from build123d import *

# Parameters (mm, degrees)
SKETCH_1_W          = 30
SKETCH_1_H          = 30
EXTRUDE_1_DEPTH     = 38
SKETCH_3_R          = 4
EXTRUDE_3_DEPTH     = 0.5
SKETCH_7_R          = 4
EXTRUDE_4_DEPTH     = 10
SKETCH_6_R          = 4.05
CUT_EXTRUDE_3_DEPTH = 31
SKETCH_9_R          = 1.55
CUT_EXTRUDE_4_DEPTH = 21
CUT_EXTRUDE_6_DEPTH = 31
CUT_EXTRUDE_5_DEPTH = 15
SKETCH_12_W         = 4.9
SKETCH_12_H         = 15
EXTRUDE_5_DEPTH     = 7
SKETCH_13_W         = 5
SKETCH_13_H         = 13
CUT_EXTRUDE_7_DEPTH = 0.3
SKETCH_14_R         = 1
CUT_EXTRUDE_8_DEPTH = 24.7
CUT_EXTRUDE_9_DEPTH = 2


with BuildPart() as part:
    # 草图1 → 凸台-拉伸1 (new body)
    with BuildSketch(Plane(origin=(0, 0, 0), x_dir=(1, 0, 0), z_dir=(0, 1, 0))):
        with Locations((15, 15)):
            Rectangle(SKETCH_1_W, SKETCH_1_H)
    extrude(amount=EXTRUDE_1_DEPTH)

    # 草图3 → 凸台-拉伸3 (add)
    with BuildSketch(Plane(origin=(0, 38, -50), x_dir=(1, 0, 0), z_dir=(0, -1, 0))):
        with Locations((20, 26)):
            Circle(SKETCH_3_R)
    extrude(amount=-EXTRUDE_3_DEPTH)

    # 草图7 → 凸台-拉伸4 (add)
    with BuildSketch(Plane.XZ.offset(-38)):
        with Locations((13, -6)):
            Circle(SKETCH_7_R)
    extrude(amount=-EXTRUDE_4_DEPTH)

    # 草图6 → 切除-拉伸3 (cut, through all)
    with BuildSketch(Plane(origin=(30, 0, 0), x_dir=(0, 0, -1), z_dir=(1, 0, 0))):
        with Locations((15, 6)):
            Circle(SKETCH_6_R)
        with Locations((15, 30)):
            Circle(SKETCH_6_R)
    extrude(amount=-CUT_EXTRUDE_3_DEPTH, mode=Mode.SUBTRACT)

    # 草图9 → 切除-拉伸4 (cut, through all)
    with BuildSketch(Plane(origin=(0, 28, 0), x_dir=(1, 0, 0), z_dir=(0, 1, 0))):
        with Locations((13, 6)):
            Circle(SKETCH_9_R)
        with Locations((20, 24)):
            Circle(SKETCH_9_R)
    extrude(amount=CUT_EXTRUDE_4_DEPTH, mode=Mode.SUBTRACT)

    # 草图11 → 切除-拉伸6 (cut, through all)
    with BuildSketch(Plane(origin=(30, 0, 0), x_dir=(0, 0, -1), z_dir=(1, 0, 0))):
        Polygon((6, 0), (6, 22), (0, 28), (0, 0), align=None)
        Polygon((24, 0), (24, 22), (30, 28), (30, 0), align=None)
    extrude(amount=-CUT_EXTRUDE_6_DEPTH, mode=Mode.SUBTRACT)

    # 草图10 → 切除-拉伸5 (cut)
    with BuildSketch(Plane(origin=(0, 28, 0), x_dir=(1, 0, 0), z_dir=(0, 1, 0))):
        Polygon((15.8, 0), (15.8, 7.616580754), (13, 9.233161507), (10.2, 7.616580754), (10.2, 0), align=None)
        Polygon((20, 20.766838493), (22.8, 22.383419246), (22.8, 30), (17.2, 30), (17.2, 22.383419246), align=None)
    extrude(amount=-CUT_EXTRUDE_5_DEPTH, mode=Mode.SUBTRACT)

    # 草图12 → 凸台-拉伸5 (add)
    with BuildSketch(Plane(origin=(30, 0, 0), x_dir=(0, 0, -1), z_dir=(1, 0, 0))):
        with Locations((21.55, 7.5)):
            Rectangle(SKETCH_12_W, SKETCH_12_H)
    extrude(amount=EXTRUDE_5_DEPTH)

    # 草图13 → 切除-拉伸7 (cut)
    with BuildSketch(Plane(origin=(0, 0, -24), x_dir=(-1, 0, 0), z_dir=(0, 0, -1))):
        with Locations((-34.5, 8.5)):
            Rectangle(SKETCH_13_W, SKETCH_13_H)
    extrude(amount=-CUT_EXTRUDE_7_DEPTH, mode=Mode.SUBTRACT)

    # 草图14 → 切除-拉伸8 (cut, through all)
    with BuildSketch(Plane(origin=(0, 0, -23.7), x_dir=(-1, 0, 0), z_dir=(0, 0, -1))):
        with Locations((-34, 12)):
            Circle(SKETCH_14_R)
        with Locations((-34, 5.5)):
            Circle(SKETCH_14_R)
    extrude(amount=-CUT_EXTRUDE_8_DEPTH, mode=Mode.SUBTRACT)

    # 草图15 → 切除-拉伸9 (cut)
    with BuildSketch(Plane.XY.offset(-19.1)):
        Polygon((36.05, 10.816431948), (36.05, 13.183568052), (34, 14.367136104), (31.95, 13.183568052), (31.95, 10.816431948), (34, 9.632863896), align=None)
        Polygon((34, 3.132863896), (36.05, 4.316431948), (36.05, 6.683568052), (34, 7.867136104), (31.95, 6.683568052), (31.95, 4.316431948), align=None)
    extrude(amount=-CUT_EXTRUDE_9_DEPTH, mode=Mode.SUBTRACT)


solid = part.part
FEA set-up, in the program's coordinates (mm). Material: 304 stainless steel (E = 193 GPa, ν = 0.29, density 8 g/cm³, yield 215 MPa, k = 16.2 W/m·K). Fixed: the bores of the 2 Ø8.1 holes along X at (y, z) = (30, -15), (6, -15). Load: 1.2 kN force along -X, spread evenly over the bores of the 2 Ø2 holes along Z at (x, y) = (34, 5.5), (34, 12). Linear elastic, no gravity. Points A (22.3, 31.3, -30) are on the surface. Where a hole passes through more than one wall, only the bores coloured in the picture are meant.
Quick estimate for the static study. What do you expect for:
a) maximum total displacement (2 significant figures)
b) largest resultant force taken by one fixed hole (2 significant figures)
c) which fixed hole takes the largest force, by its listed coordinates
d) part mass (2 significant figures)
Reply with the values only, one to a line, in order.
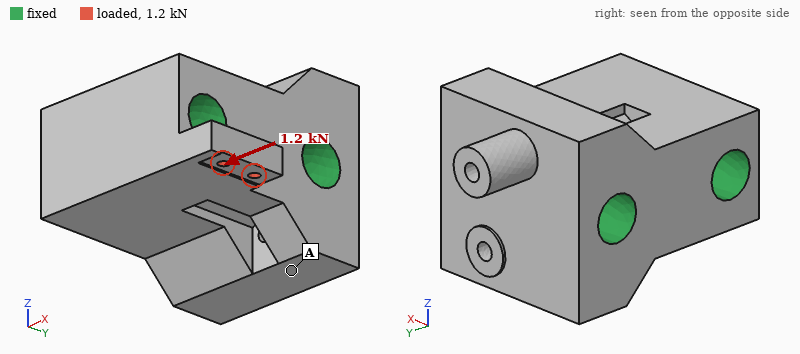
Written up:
3.6 µm
1.1 kN
(6, -15)
180 g
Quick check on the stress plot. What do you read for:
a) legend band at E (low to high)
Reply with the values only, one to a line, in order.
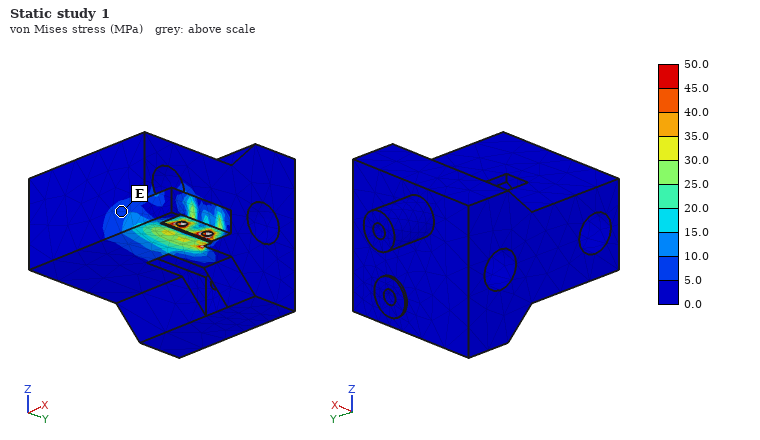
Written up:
5.0 to 10.0 MPa
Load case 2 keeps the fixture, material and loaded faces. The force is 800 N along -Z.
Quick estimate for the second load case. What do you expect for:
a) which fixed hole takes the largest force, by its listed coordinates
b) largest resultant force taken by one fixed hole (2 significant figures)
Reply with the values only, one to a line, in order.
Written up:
(6, -15)
750 N
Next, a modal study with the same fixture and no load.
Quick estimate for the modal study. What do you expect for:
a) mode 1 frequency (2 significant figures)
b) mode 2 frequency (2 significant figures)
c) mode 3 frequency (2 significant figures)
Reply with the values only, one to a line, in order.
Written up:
30 kHz
32 kHz
40 kHz
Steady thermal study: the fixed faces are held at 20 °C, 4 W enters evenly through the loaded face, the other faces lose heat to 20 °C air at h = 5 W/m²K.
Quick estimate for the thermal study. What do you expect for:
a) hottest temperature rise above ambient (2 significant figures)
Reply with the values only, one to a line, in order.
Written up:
39 K
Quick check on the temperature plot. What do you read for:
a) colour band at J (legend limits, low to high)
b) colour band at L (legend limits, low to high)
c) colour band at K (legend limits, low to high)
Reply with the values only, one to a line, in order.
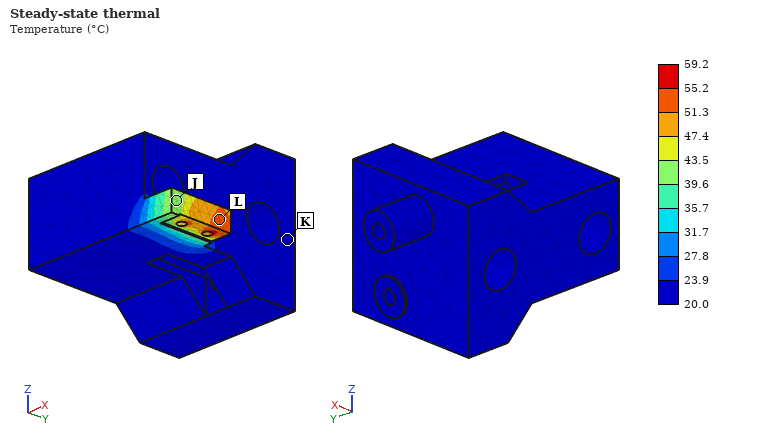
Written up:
39.6 to 43.5 °C
51.3 to 55.2 °C
20.0 to 23.9 °C
